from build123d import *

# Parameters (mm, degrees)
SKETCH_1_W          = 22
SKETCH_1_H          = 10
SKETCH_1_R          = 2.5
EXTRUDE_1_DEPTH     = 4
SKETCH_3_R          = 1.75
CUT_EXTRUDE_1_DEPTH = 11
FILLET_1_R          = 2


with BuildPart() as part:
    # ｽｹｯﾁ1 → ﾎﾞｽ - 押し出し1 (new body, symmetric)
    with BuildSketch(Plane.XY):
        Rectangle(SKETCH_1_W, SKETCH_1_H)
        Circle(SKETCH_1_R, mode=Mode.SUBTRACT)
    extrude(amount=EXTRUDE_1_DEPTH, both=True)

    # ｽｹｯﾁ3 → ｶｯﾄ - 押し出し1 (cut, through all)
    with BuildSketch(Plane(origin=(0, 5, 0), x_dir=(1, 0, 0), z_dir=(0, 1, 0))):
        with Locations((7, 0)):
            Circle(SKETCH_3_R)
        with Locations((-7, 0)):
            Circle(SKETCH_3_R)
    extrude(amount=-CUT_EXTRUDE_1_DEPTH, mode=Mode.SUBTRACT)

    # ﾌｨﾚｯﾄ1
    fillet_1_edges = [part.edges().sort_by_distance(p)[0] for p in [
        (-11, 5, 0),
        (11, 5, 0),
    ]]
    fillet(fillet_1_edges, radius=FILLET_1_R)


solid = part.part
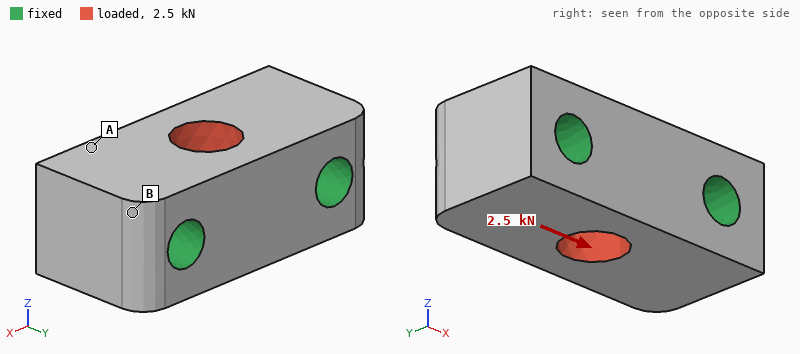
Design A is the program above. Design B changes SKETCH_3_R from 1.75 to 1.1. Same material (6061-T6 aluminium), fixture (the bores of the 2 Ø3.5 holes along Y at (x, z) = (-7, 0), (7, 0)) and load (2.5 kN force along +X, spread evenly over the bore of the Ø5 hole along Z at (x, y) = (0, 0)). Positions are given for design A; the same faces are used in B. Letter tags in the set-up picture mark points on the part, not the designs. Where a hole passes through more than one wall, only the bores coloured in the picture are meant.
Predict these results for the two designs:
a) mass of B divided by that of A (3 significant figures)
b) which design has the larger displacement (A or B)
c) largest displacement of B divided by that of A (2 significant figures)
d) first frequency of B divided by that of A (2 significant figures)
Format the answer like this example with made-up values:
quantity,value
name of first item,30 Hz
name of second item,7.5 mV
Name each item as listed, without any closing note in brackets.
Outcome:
quantity,value
mass of B divided by that of A,1.08
which design has the larger displacement,B
largest displacement of B divided by that of A,1.2
first frequency of B divided by that of A,0.74
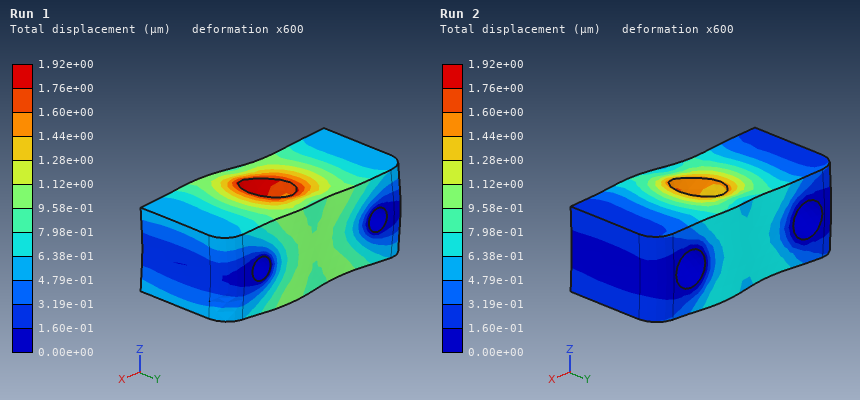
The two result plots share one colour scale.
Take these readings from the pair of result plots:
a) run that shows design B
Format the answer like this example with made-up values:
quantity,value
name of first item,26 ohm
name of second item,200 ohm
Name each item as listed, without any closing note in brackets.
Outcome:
quantity,value
run that shows design B,Run 1
